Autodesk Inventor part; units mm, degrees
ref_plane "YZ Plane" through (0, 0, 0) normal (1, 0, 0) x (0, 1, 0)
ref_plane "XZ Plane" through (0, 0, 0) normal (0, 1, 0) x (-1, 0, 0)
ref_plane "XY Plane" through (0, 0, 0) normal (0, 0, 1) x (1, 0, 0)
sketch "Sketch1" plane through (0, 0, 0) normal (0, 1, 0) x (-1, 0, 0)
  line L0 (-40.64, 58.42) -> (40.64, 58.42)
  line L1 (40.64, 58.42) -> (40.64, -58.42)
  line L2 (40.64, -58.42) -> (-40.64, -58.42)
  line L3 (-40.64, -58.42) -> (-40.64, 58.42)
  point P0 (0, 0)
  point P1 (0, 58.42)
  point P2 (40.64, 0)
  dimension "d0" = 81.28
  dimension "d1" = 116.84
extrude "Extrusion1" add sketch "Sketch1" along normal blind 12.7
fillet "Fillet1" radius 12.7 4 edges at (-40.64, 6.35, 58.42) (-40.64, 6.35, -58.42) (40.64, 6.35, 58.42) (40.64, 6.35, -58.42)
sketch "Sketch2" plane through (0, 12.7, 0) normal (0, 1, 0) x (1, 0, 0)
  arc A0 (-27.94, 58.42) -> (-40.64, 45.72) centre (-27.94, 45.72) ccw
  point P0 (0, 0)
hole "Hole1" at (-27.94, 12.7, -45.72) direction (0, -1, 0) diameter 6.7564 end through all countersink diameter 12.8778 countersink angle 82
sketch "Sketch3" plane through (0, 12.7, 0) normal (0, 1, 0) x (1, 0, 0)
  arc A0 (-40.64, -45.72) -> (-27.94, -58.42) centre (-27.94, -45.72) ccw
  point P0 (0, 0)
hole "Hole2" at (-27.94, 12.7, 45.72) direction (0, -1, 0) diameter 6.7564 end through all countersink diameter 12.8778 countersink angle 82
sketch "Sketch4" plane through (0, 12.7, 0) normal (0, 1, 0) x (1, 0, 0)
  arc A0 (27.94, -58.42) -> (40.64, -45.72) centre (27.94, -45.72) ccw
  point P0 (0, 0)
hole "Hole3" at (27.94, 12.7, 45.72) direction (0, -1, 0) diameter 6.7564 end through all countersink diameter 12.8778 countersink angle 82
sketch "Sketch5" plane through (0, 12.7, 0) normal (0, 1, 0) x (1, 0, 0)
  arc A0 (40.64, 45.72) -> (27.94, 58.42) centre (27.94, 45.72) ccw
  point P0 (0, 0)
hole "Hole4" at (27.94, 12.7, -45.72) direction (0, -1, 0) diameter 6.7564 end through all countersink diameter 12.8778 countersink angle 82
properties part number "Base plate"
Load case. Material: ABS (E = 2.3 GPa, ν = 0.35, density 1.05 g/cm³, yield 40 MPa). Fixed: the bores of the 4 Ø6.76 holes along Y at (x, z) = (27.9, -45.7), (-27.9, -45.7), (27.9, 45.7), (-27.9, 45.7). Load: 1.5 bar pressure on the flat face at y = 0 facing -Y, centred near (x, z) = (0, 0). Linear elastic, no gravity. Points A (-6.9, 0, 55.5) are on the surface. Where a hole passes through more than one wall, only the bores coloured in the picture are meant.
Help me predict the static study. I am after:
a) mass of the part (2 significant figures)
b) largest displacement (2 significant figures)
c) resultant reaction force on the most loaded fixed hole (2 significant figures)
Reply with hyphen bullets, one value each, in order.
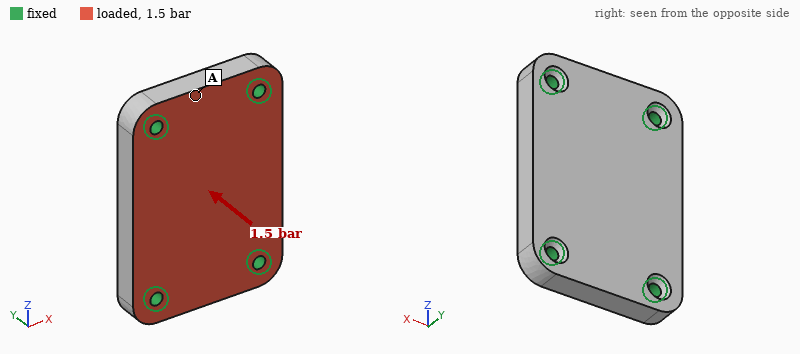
- 120 g
- 0.13 mm
- 350 N
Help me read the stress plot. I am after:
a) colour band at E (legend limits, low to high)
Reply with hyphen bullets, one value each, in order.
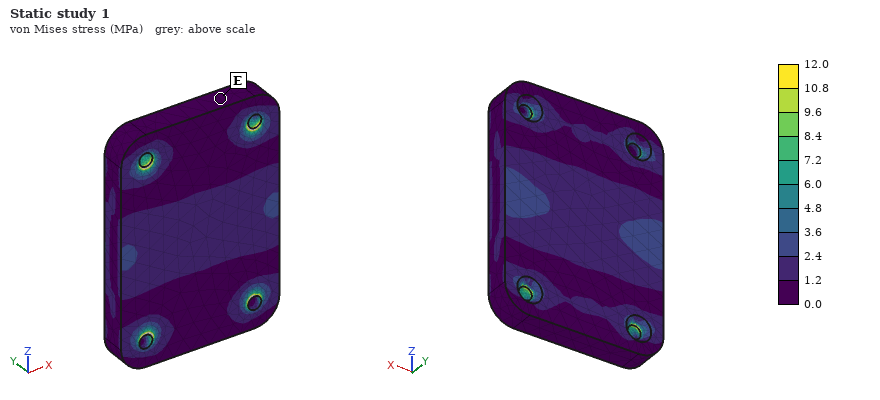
- 0.0 to 1.2 MPa
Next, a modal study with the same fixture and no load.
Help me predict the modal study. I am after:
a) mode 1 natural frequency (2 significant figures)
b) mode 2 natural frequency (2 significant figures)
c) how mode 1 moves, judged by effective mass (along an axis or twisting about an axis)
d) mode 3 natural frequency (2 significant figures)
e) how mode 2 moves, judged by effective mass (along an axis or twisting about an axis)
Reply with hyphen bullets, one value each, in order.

- 1600 Hz
- 2300 Hz
- along Y
- 3600 Hz
- twisting about Z
